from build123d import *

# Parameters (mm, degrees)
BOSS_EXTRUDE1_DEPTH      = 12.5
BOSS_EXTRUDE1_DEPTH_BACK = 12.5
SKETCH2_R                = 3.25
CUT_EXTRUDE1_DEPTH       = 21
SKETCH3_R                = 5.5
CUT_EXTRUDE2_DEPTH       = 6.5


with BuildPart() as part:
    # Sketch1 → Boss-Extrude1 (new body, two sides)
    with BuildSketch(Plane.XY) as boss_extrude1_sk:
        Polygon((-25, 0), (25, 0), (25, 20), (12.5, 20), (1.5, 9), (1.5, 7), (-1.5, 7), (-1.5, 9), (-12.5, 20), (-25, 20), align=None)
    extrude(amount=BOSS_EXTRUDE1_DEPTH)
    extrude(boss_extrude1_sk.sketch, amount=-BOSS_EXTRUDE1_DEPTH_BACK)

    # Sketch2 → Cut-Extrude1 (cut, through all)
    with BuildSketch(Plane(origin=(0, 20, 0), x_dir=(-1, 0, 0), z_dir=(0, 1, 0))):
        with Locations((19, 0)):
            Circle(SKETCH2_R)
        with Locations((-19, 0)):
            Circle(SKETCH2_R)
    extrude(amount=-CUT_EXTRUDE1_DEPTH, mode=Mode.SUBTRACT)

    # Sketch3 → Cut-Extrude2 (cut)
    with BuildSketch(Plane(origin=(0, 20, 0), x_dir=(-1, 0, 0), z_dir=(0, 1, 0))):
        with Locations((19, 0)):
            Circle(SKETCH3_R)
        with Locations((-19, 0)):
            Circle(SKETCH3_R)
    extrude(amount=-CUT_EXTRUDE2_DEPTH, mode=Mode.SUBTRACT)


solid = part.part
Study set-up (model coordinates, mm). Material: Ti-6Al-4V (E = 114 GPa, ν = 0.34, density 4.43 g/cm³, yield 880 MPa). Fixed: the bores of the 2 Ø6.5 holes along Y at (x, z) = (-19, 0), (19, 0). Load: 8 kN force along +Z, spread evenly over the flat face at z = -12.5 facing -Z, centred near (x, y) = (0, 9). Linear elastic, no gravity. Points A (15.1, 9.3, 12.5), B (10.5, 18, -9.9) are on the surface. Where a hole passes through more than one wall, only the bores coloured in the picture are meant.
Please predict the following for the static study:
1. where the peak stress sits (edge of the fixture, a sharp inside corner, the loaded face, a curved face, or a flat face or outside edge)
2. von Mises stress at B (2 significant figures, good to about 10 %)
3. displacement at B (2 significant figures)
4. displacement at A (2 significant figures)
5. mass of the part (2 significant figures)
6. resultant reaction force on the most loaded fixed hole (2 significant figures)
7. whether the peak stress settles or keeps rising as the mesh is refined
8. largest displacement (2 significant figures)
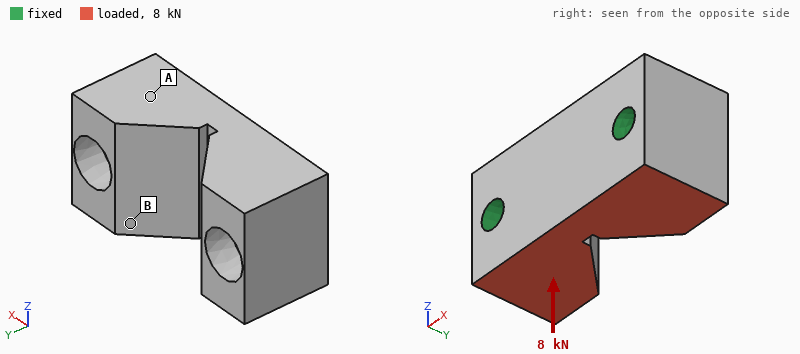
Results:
edge of the fixture
13 MPa
3.8 µm
1.7 µm
84 g
4.0 kN
keeps rising
4.5 µm
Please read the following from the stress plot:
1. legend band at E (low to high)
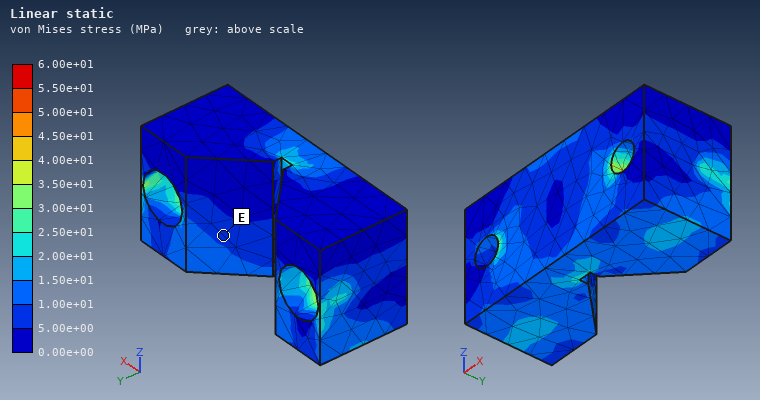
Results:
5.00e+00 to 1.00e+01 MPa
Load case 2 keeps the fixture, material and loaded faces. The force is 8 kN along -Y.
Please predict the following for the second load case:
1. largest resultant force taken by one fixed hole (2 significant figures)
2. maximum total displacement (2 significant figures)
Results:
4.0 kN
15 µm
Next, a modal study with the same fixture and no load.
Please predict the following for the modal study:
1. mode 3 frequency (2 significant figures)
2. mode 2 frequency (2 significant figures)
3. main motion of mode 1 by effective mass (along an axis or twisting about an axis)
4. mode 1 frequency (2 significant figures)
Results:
28 kHz
27 kHz
along Y
25 kHz
